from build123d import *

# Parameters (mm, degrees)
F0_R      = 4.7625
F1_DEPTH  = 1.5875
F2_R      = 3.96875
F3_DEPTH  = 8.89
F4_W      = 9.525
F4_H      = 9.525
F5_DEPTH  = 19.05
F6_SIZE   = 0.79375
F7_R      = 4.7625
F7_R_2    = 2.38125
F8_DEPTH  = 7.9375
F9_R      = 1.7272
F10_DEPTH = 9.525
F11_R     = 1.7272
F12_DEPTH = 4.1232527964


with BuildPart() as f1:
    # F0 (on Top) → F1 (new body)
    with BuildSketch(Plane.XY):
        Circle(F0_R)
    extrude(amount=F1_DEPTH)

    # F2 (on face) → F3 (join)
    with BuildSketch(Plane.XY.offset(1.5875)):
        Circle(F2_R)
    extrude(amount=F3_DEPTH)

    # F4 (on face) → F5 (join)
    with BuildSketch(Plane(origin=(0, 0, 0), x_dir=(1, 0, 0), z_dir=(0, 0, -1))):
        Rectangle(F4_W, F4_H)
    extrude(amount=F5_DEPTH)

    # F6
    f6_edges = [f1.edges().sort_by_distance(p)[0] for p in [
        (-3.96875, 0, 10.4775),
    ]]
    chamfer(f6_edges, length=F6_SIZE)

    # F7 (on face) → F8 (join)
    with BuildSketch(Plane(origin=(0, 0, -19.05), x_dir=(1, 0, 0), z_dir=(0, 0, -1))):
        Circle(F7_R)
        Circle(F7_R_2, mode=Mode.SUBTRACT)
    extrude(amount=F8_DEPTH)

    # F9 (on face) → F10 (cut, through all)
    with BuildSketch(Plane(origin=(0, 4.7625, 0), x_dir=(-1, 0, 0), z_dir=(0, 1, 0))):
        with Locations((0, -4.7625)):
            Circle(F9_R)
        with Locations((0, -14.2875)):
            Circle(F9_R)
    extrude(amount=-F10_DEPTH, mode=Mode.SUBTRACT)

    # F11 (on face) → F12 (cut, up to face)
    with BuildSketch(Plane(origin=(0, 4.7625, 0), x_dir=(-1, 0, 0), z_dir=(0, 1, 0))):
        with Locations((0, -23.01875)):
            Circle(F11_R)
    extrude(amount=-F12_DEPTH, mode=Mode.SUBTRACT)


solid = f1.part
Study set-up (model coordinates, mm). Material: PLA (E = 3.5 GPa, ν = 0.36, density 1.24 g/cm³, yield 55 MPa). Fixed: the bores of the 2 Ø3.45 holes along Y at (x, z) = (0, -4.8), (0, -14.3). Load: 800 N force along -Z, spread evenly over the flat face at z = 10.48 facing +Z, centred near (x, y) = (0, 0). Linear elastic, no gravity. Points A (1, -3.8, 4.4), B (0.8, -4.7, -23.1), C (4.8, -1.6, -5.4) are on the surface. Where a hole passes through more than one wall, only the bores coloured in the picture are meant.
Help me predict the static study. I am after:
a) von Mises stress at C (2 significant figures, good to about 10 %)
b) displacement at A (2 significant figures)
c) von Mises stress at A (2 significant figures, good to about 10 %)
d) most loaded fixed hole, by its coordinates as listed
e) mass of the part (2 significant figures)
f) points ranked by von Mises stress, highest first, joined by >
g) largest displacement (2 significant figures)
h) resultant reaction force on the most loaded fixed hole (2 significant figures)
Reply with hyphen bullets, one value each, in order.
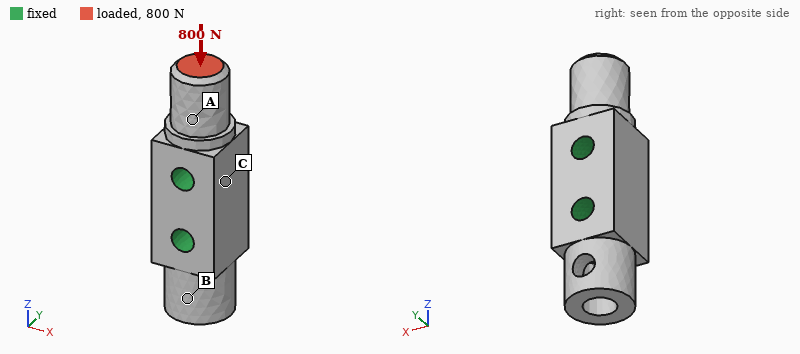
- 4.6 MPa
- 32 µm
- 16 MPa
- (0, -4.8)
- 3.1 g
- A > C > B
- 68 µm
- 730 N
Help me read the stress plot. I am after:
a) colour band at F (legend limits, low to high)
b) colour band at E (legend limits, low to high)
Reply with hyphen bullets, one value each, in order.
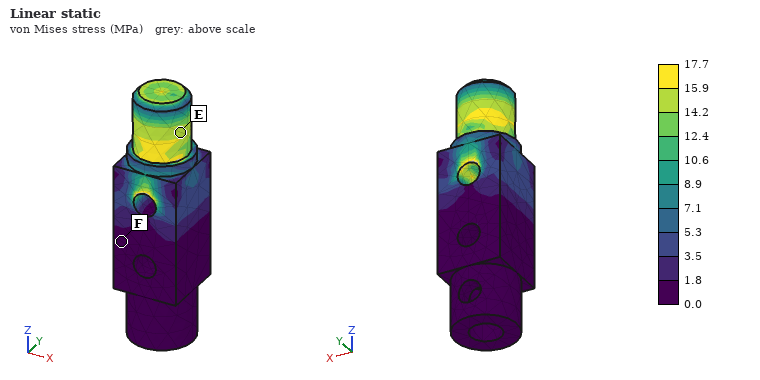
- 0.0 to 1.8 MPa
- 14.2 to 15.9 MPa
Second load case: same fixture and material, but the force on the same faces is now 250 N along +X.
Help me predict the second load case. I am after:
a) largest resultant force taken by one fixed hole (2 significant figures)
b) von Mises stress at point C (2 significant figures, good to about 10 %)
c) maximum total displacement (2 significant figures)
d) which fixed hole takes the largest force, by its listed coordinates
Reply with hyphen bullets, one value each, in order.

- 400 N
- 17 MPa
- 0.33 mm
- (0, -4.8)
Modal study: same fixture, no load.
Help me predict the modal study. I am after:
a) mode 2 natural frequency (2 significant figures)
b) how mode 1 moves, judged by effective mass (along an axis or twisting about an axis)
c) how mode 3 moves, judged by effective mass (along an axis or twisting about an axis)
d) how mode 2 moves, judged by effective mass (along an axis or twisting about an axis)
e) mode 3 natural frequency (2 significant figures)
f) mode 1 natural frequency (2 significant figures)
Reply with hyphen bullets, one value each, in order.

- 11 kHz
- along X
- along X
- along Y
- 12 kHz
- 9400 Hz
